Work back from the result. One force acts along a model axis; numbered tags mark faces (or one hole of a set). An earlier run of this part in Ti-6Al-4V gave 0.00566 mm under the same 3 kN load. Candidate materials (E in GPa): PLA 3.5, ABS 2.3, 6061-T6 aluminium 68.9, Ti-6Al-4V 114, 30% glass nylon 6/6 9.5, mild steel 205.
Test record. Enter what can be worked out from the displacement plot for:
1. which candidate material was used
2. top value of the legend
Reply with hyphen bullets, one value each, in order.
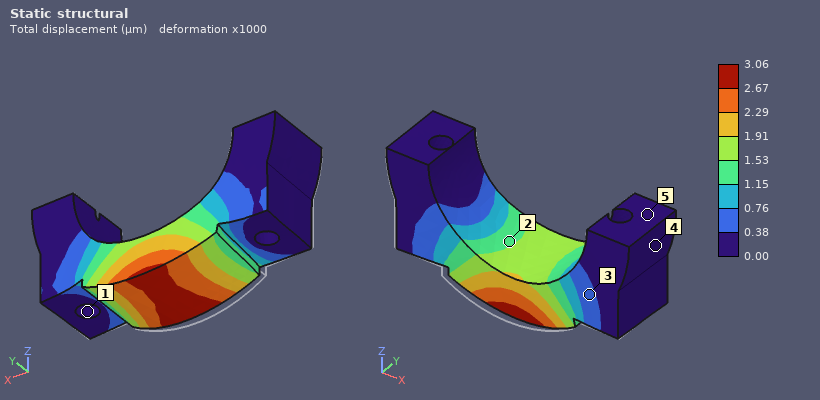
- mild steel
- 3.06 µm
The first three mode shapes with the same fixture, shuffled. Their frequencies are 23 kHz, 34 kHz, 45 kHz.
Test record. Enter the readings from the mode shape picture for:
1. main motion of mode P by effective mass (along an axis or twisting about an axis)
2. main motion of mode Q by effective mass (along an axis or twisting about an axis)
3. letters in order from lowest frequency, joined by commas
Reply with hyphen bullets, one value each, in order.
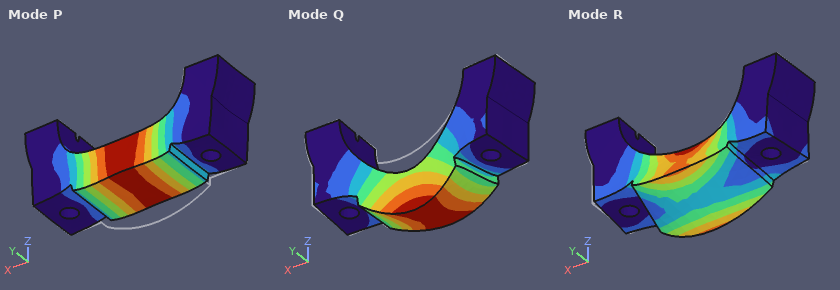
- along Z
- along Y
- Q, P, R
